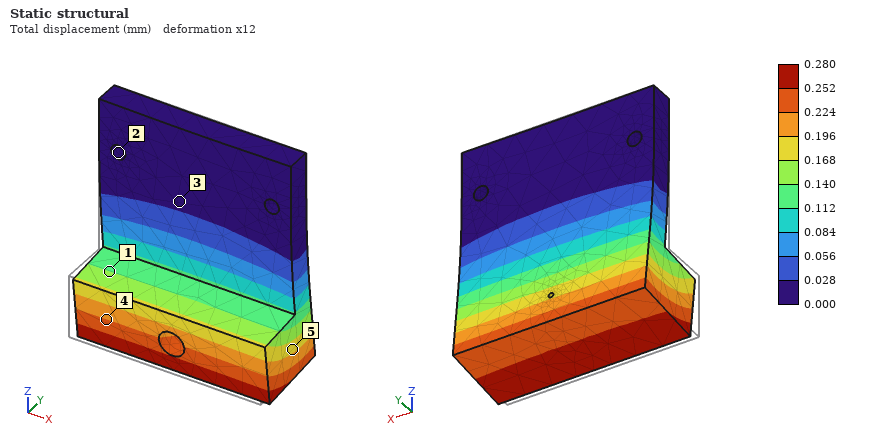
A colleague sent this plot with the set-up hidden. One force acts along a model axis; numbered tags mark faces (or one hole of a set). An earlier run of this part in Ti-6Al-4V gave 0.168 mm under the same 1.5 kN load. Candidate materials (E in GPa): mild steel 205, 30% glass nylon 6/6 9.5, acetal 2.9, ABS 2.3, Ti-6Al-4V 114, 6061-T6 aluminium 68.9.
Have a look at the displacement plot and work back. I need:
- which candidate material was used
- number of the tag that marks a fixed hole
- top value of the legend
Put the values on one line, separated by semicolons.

6061-T6 aluminium; 2; 0.280 mm
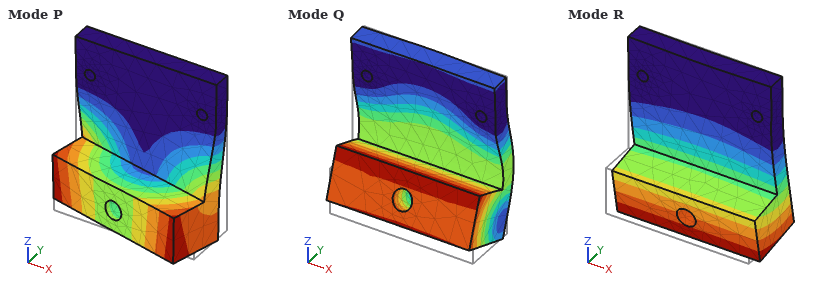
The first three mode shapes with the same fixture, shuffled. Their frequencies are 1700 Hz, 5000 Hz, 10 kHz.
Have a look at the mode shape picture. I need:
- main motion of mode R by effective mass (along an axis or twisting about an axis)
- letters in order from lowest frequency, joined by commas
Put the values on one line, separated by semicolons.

along Y; R, P, Q
